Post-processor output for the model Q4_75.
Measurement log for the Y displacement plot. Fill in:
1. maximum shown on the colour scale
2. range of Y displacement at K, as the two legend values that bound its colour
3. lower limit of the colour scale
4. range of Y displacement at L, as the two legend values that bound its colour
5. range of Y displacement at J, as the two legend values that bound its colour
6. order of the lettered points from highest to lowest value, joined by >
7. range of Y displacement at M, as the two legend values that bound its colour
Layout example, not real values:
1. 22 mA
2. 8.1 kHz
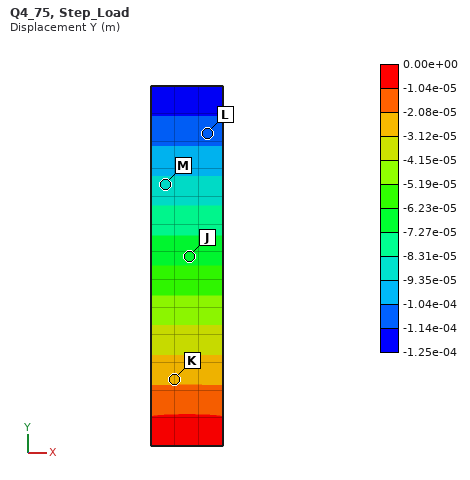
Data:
1. 0.00e+00 m
2. -3.12e-05 to -2.08e-05 m
3. -1.25e-04 m
4. -1.14e-04 to -1.04e-04 m
5. -7.27e-05 to -6.23e-05 m
6. K > J > M > L
7. -9.35e-05 to -8.31e-05 m
